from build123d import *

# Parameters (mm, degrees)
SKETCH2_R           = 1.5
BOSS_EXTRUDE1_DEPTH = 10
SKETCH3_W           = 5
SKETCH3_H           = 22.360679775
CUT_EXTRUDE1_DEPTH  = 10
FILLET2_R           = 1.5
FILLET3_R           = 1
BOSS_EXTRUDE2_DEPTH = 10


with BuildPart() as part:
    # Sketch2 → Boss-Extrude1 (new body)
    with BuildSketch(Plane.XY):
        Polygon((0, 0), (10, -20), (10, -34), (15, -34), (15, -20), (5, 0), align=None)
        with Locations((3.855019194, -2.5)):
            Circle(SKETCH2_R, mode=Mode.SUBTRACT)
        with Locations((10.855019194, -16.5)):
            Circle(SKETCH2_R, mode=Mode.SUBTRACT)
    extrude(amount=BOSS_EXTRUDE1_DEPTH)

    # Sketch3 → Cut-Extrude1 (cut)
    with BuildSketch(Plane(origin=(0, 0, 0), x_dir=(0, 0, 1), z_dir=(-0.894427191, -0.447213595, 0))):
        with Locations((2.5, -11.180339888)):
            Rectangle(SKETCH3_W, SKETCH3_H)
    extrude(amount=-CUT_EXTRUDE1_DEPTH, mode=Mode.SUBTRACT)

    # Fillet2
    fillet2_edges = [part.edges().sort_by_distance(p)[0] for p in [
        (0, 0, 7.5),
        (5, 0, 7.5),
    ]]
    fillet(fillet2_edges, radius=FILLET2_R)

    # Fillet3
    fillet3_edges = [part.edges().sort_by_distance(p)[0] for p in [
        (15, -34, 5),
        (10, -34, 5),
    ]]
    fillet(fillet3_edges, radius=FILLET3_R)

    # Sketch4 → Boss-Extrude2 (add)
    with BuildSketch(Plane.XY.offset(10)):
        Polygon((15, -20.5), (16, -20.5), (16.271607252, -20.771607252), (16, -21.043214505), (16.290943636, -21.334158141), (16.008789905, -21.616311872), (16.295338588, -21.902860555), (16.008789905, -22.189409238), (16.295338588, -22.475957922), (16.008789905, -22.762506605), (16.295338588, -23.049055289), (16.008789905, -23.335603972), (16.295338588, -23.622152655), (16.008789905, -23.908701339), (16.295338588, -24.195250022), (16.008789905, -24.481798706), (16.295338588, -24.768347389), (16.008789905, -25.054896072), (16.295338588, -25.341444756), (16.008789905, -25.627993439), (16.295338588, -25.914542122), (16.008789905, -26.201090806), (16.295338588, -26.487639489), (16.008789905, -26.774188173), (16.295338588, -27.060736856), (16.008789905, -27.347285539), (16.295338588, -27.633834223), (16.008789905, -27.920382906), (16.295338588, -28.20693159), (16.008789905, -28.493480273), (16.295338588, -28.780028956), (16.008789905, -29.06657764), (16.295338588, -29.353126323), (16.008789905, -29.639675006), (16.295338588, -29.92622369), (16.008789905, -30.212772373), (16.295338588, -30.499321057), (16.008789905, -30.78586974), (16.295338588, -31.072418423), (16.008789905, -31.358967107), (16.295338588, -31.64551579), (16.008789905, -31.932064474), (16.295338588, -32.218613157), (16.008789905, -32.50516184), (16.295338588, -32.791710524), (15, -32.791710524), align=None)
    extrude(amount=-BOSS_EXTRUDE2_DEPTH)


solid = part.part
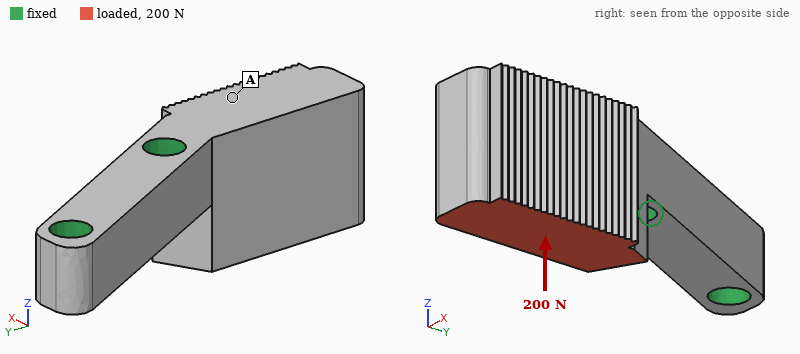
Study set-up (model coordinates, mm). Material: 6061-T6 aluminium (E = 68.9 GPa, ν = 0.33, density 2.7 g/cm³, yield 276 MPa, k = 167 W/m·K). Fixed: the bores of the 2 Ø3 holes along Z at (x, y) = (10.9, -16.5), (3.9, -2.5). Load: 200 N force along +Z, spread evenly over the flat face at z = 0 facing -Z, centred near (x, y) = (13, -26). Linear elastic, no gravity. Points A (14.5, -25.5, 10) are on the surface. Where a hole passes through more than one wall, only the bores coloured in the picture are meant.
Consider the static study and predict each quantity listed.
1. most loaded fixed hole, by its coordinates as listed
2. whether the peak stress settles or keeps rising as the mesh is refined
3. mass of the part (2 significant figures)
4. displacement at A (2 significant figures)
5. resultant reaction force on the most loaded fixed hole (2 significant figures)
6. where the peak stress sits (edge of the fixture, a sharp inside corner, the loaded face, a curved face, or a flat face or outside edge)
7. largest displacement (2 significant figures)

(10.9, -16.5)
keeps rising
3.5 g
15 µm
200 N
edge of the fixture
33 µm
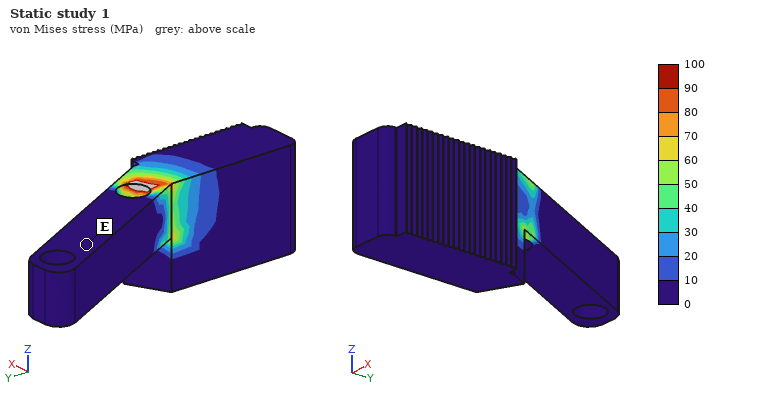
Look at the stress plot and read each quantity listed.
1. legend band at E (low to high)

0 to 10 MPa
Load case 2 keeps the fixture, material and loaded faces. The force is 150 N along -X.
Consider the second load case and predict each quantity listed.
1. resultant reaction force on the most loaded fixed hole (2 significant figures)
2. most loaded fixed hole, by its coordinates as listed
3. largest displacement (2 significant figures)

150 N
(10.9, -16.5)
48 µm
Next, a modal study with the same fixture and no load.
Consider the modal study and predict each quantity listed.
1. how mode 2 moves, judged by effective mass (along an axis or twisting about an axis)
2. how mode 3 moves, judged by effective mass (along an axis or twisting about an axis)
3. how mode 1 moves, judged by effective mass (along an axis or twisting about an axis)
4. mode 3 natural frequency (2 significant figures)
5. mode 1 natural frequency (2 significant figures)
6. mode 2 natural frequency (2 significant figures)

along Z
twisting about Y
along X
21 kHz
8200 Hz
9600 Hz
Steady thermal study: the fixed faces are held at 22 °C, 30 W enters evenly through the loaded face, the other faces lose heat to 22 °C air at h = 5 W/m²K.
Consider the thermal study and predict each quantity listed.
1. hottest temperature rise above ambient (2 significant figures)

55 K
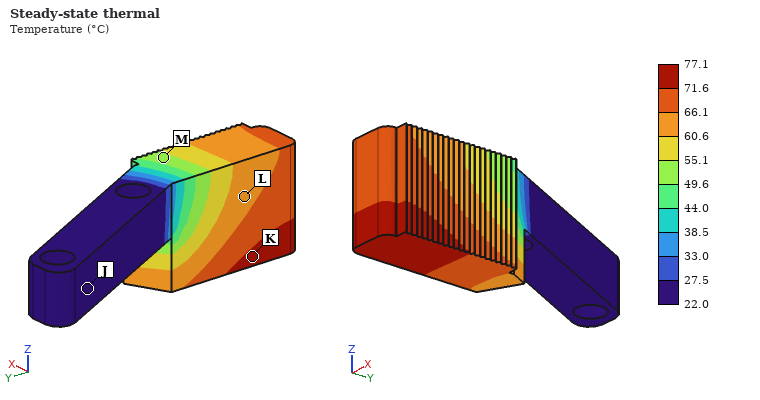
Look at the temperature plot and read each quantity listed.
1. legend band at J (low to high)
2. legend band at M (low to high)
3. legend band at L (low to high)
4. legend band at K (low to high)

22.0 to 27.5 °C
49.6 to 55.1 °C
60.6 to 66.1 °C
71.6 to 77.1 °C
